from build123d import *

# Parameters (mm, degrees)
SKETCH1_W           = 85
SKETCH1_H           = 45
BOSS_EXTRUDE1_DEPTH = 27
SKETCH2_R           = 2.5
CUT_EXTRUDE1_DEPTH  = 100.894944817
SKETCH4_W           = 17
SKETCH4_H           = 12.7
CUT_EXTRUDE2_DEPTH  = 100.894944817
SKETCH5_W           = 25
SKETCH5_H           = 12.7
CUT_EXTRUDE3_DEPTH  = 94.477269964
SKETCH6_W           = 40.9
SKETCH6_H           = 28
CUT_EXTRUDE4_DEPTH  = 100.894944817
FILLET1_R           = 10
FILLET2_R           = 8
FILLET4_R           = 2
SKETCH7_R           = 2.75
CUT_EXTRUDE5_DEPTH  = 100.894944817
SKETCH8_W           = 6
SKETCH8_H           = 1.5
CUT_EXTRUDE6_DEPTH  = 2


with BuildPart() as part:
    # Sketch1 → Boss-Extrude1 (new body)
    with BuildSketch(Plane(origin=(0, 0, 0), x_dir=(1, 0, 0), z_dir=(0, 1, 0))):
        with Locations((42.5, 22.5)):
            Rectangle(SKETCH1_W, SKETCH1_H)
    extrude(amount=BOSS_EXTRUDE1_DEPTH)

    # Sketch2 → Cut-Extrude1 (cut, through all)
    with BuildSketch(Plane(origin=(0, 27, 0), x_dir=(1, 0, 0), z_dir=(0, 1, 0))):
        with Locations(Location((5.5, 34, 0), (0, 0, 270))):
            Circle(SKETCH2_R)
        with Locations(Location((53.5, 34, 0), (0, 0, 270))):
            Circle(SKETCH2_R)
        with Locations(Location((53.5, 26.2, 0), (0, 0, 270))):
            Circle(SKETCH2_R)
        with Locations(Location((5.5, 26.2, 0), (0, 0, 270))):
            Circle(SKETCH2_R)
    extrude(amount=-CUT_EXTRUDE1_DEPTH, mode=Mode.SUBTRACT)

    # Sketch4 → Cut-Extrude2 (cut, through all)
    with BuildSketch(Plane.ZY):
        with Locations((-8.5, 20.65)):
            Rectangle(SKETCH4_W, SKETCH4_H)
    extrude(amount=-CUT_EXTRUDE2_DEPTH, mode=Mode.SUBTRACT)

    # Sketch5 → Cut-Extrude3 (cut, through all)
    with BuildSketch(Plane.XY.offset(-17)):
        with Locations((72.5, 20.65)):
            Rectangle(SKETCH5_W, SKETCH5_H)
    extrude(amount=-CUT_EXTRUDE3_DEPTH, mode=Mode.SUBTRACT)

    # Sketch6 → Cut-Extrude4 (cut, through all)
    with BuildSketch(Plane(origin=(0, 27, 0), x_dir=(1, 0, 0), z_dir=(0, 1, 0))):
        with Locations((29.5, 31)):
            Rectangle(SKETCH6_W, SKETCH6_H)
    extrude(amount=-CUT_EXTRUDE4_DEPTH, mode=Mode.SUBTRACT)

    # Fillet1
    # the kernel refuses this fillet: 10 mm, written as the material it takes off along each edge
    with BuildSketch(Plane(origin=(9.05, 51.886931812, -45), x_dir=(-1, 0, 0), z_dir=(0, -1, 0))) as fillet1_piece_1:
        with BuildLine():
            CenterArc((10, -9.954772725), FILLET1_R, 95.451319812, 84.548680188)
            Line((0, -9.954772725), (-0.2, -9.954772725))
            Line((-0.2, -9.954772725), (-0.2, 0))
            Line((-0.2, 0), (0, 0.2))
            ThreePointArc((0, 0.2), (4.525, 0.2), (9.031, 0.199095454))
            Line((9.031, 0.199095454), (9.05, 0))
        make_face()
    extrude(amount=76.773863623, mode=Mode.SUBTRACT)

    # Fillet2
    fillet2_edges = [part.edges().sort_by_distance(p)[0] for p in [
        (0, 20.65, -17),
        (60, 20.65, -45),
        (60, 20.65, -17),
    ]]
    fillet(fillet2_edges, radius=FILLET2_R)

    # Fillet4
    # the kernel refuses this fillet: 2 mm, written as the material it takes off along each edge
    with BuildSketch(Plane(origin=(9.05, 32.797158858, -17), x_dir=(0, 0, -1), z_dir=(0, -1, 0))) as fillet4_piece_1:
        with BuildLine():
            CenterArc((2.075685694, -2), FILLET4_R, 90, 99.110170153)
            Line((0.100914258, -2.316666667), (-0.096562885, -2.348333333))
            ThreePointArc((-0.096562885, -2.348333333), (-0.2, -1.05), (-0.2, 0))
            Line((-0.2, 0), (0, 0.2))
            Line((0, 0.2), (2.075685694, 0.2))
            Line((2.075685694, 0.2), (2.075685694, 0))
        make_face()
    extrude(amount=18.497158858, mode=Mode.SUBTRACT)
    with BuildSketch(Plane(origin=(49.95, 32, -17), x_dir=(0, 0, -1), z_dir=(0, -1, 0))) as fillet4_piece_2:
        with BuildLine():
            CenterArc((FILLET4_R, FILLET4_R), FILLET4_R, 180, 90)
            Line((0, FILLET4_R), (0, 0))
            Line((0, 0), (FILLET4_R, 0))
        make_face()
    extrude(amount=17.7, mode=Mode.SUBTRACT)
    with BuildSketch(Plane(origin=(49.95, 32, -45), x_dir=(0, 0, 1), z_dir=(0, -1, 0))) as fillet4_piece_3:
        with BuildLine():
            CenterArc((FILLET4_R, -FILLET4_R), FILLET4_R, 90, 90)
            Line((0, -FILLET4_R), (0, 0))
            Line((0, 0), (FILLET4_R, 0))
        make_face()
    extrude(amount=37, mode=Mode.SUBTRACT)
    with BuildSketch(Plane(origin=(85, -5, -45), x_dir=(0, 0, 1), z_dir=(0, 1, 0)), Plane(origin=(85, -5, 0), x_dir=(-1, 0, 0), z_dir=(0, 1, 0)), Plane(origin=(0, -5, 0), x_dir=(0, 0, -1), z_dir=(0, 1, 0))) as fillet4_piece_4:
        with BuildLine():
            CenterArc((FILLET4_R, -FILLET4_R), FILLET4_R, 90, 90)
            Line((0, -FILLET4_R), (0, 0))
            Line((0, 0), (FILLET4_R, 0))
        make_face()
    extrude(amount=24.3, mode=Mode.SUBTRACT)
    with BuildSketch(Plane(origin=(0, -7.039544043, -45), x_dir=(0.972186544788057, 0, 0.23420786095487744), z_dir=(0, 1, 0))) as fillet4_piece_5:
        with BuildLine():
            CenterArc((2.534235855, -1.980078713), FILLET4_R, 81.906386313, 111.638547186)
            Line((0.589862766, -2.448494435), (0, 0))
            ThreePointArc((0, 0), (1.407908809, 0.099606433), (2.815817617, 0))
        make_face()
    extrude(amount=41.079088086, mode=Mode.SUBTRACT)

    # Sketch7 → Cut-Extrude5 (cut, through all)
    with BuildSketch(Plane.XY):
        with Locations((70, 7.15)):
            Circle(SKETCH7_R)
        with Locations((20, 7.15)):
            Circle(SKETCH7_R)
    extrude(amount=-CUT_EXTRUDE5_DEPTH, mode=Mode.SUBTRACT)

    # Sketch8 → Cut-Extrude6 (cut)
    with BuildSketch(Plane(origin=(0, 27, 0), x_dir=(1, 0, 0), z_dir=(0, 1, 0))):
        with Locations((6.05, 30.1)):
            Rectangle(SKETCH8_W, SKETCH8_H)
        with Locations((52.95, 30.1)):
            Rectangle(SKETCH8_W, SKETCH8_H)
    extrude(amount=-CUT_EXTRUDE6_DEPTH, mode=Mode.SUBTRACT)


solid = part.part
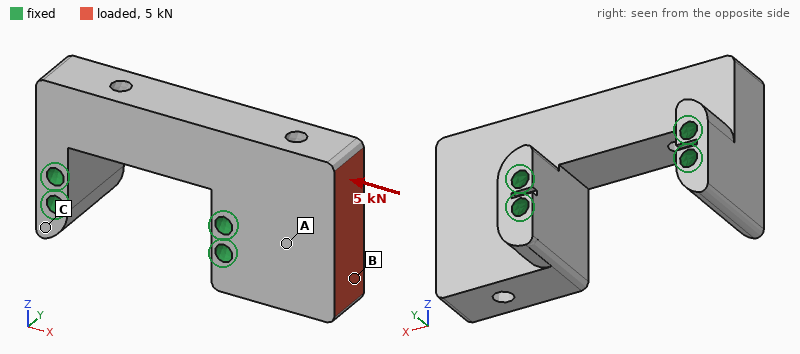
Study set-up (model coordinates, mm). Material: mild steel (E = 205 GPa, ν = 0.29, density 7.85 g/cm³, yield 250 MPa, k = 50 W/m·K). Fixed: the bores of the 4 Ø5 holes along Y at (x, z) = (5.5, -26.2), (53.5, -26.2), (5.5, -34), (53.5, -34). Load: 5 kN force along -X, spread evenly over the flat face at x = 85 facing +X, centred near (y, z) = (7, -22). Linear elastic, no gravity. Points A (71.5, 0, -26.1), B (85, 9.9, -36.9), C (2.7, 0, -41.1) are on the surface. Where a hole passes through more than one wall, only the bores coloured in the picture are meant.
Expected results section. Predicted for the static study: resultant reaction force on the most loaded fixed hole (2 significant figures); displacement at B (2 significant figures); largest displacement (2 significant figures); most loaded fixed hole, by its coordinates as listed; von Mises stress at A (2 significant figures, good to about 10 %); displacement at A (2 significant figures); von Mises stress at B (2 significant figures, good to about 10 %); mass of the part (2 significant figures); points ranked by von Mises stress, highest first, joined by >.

3.4 kN
2.3 µm
4.3 µm
(53.5, -26.2)
12 MPa
1.8 µm
7.0 MPa
320 g
A > B > C
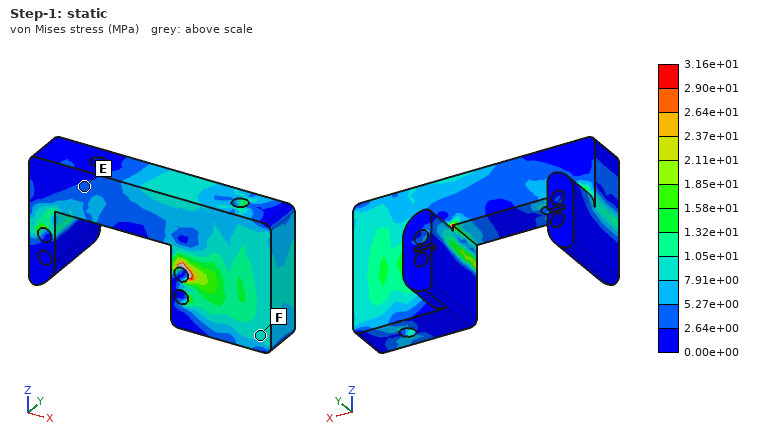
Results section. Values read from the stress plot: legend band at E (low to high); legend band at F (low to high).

2.64e+00 to 5.27e+00 MPa
7.91e+00 to 1.05e+01 MPa
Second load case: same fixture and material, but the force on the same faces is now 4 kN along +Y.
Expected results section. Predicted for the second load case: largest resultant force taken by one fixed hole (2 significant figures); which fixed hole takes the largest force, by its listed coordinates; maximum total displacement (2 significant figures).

3.2 kN
(53.5, -26.2)
30 µm
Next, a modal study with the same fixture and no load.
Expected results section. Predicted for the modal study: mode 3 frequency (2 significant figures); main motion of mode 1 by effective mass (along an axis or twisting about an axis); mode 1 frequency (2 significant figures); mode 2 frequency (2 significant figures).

10 kHz
along Y
8900 Hz
9900 Hz
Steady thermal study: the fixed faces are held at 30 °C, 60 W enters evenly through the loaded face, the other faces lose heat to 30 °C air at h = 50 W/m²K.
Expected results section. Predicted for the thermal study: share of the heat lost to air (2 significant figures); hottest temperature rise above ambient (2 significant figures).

16 %
69 K
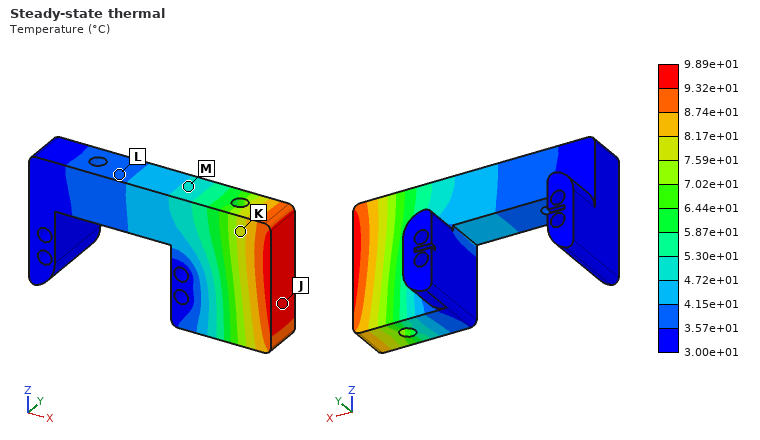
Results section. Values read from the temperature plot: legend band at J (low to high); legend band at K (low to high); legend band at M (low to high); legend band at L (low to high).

9.32e+01 to 9.89e+01 °C
7.59e+01 to 8.17e+01 °C
4.72e+01 to 5.30e+01 °C
3.57e+01 to 4.15e+01 °C
